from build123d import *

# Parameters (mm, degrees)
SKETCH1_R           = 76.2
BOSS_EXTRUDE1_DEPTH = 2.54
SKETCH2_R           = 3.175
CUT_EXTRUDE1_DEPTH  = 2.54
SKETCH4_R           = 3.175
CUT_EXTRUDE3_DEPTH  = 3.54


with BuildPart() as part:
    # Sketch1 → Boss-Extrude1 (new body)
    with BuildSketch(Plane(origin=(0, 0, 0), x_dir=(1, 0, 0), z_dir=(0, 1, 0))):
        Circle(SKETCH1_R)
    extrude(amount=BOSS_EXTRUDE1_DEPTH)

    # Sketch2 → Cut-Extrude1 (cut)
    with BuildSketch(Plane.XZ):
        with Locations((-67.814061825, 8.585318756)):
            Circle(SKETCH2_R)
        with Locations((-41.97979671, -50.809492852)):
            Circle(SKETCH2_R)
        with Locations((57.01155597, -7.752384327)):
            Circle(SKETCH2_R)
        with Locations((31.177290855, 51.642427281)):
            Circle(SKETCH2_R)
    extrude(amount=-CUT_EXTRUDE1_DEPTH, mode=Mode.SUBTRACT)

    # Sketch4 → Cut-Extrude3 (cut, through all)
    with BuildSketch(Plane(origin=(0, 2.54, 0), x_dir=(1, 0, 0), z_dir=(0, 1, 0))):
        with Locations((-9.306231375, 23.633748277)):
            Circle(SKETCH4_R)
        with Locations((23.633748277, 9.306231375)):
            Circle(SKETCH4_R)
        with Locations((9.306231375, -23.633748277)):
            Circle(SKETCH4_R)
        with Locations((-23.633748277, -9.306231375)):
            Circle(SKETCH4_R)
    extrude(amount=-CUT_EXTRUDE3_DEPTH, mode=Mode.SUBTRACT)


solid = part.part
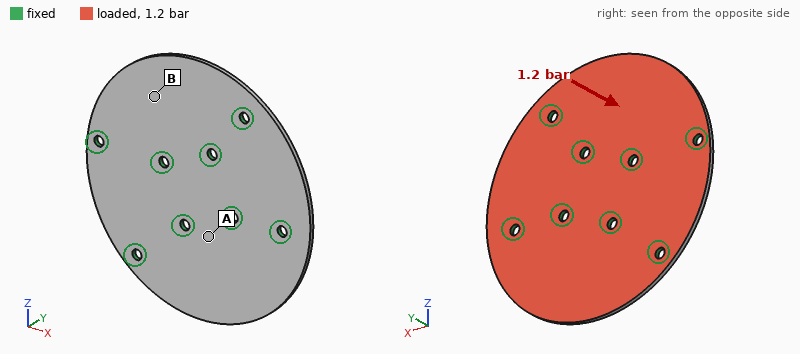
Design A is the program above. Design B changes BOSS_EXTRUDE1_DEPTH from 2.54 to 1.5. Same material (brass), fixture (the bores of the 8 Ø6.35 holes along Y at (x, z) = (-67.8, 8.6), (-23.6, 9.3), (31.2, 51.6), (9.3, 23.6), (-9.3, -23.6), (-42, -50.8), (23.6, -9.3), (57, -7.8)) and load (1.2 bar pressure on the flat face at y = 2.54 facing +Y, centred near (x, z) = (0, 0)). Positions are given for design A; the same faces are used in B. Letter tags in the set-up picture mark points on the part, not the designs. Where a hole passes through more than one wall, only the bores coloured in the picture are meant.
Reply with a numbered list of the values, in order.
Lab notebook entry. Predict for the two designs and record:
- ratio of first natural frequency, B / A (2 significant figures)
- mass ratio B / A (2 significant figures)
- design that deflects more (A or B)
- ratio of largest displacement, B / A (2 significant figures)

1. 0.60
2. 0.59
3. B
4. 4.8
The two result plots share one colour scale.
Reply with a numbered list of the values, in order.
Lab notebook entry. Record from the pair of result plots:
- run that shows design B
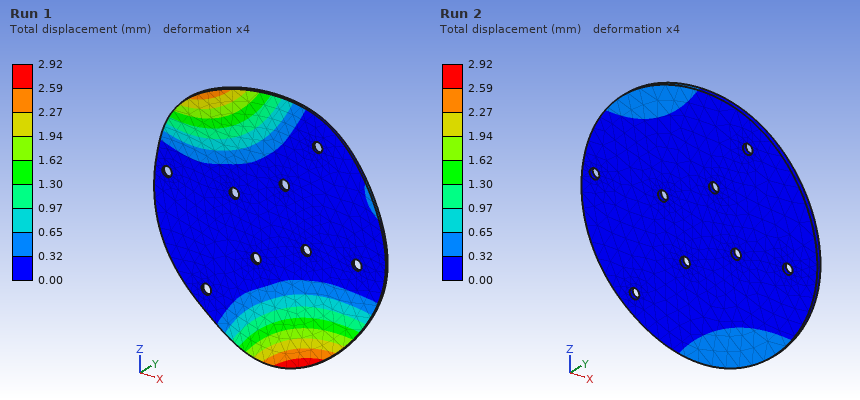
1. Run 1
